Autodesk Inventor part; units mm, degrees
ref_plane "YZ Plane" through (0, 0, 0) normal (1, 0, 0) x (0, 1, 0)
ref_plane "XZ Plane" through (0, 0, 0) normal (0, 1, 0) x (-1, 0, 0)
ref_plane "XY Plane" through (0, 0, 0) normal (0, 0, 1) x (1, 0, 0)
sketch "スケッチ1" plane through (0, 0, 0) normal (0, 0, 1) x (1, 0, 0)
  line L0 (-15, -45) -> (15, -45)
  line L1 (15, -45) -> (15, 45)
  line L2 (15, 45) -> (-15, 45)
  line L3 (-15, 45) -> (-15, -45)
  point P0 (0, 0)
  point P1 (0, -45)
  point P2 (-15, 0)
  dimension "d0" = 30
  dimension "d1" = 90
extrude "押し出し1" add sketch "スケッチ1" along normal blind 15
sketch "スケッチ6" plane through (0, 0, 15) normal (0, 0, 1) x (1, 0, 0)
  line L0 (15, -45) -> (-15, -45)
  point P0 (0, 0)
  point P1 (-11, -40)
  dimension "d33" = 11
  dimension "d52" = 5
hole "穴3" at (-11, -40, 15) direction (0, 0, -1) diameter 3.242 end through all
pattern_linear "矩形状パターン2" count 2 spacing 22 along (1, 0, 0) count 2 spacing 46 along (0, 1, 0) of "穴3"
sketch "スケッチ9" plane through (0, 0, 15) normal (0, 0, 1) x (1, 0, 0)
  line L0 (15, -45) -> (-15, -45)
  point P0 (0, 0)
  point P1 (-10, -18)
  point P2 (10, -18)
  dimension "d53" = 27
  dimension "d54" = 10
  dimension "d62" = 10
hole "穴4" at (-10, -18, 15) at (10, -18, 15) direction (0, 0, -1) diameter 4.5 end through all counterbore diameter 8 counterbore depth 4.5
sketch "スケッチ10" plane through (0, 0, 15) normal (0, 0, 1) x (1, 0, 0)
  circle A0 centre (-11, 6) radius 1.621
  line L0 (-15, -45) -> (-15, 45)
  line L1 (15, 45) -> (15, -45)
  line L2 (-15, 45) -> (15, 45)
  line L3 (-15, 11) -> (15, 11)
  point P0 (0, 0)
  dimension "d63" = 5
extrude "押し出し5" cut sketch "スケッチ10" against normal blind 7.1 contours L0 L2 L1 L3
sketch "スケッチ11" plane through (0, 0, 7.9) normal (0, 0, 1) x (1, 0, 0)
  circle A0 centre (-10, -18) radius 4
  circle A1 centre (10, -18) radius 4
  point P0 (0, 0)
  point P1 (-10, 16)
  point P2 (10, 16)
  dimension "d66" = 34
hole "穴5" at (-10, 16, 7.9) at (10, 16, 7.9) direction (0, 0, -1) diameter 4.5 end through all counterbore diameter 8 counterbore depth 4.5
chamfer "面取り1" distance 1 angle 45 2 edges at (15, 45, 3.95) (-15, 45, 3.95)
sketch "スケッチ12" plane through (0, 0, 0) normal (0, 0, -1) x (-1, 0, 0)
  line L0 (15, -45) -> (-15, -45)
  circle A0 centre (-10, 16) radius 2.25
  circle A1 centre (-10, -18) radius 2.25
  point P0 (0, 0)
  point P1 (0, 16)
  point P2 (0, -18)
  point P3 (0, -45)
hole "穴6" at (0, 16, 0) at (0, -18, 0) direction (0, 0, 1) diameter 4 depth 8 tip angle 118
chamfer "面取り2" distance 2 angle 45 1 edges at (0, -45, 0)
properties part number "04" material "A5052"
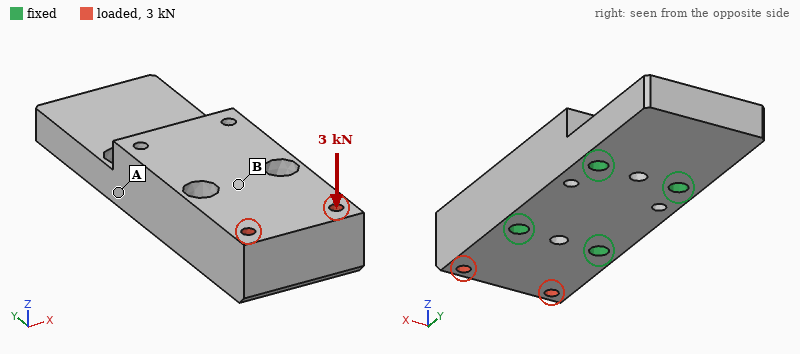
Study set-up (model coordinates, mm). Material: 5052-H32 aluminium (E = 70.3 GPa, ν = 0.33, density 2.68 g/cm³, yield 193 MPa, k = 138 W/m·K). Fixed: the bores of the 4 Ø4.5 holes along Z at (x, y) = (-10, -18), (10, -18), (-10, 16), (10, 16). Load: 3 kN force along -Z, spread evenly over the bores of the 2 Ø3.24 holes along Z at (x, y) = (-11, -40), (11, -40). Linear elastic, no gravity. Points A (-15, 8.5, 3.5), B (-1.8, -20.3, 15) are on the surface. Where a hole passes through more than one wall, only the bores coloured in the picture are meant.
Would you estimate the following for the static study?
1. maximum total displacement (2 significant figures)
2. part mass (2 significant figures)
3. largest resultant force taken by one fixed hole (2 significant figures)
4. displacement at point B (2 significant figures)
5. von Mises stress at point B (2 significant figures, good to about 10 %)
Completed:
50 µm
83 g
1.9 kN
9.4 µm
45 MPa
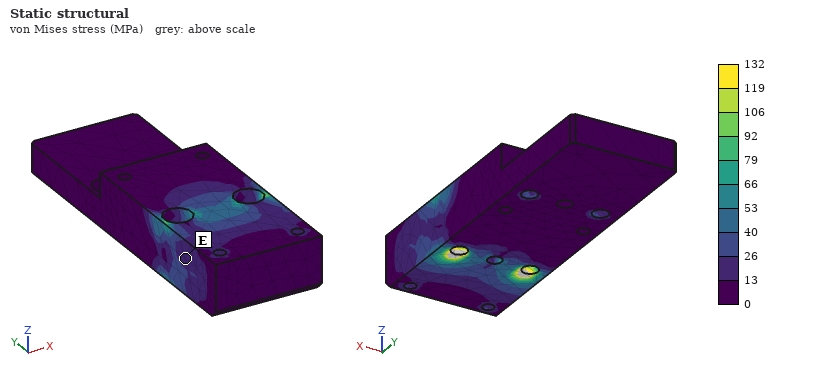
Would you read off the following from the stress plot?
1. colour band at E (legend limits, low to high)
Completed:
13 to 26 MPa
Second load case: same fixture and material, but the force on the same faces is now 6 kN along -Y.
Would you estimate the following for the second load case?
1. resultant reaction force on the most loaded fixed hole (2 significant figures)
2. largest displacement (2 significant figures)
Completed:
2.8 kN
10 µm
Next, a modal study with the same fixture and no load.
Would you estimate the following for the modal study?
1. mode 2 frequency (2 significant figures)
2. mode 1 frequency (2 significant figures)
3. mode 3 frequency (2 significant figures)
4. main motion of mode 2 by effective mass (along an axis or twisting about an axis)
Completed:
11 kHz
5500 Hz
13 kHz
along Z
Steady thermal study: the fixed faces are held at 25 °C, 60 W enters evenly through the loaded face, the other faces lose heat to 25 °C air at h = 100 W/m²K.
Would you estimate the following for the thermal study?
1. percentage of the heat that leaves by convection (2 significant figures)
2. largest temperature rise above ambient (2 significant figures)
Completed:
7.7 %
26 K
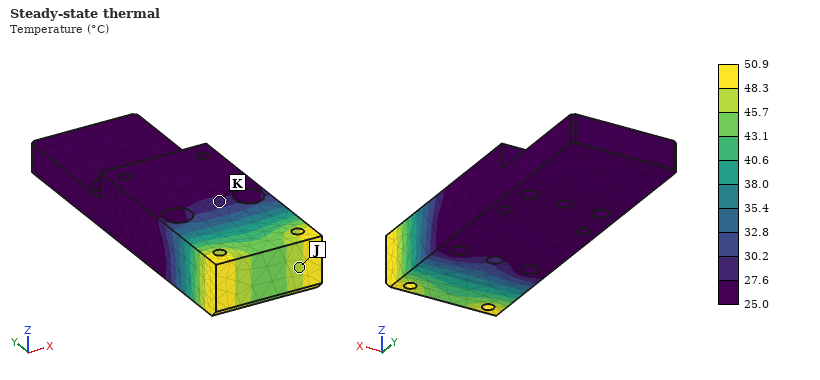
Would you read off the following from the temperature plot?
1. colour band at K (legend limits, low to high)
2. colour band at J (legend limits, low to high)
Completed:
27.6 to 30.2 °C
45.7 to 48.3 °C
